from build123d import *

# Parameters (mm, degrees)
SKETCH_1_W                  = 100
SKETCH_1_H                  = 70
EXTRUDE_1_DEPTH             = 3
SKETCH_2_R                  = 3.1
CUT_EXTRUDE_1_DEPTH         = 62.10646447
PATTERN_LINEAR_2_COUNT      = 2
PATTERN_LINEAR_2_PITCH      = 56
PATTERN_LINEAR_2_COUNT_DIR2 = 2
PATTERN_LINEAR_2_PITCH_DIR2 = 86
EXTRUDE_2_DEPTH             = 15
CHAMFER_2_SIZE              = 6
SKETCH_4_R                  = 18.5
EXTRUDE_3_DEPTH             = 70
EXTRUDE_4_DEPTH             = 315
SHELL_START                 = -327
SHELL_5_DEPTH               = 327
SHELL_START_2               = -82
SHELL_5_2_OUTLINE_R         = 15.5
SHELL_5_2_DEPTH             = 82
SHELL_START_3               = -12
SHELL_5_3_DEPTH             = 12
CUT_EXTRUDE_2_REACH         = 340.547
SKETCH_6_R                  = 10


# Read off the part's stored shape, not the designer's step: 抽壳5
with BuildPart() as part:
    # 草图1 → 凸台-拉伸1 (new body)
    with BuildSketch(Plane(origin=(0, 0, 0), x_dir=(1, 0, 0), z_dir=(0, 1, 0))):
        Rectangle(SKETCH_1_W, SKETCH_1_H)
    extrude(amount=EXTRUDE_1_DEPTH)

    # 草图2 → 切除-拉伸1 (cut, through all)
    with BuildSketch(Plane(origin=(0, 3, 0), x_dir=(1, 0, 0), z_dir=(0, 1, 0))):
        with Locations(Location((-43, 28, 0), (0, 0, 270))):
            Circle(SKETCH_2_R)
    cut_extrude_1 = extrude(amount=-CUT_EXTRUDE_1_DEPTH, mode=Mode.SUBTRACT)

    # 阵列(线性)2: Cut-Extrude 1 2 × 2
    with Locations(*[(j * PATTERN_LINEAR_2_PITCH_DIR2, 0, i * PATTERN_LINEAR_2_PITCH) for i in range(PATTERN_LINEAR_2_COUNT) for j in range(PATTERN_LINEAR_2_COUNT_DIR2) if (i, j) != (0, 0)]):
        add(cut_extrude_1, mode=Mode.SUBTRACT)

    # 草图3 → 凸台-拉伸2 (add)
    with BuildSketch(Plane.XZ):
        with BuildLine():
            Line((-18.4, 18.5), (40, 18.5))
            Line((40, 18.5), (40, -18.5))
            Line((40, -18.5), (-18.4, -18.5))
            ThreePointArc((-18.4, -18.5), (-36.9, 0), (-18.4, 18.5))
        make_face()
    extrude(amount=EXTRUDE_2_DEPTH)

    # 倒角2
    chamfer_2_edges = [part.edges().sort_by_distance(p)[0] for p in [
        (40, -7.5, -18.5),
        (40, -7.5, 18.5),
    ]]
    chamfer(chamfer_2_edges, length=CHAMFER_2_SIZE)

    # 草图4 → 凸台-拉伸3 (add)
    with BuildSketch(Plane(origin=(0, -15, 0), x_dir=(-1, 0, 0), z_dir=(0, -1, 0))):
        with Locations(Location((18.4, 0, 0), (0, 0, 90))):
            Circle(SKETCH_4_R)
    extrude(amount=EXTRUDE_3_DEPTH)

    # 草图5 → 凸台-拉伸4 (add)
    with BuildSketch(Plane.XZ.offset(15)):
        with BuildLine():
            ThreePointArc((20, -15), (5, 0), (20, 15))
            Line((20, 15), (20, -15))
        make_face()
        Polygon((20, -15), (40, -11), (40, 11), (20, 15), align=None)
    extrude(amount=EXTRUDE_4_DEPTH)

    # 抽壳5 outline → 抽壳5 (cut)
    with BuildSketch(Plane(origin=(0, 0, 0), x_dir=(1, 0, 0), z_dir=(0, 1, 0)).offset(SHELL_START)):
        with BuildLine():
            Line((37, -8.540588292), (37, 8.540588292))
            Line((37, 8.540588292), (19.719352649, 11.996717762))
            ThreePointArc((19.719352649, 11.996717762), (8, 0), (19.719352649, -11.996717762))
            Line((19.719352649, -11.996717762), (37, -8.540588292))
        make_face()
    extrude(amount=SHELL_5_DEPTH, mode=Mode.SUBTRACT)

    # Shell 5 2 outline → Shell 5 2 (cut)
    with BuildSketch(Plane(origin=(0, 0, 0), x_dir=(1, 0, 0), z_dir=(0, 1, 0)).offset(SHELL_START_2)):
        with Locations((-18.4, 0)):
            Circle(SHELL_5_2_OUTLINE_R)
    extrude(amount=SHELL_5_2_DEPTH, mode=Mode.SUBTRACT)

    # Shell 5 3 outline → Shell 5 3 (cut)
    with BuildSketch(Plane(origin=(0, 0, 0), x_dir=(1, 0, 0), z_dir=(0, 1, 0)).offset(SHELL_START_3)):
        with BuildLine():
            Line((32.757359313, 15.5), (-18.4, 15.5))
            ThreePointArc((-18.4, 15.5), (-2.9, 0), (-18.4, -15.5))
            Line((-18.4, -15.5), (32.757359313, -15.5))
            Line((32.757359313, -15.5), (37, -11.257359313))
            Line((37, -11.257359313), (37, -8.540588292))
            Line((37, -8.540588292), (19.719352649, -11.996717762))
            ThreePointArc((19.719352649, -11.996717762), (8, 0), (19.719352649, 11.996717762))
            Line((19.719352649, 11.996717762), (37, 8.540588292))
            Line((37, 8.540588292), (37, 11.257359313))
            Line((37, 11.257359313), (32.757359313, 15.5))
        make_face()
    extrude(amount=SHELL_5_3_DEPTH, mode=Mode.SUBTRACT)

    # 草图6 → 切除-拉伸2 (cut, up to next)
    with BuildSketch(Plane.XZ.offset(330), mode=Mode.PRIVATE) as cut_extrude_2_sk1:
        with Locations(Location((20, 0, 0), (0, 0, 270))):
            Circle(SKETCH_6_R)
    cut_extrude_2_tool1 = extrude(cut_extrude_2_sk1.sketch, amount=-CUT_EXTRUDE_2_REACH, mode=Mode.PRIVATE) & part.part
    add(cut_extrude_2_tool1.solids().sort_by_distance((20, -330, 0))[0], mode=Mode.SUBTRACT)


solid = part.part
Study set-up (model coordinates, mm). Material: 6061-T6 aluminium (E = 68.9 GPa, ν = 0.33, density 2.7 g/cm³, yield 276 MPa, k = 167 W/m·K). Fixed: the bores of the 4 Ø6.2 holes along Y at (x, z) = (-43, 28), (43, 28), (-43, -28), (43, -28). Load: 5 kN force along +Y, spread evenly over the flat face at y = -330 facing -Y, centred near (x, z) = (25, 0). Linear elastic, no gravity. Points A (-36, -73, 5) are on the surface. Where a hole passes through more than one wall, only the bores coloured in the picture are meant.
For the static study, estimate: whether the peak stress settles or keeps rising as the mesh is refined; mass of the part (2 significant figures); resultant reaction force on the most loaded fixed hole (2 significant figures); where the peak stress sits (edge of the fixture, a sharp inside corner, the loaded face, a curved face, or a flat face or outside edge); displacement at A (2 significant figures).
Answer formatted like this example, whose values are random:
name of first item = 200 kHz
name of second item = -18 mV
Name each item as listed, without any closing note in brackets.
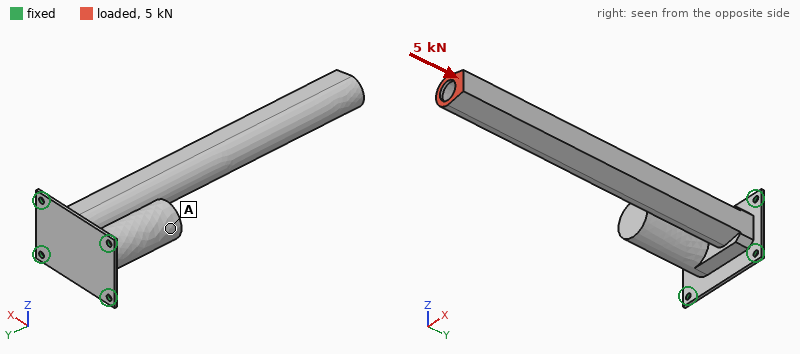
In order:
whether the peak stress settles or keeps rising as the mesh is refined = keeps rising
mass of the part = 410 g
resultant reaction force on the most loaded fixed hole = 2.2 kN
where the peak stress sits = edge of the fixture
displacement at A = 0.17 mm
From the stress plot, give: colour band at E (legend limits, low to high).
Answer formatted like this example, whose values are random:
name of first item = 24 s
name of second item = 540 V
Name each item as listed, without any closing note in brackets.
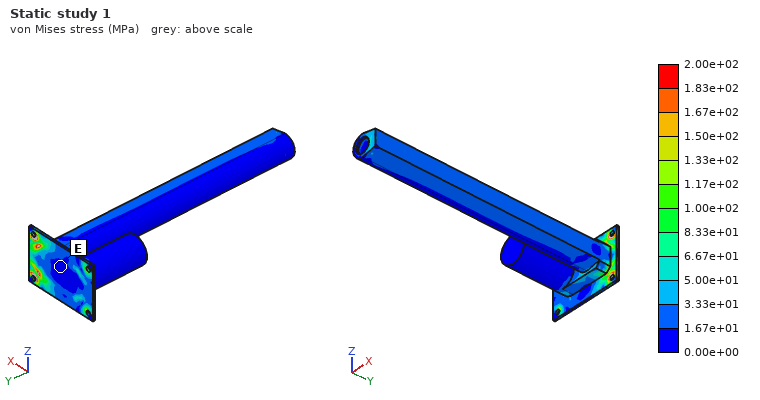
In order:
colour band at E = 0.00e+00 to 1.67e+01 MPa
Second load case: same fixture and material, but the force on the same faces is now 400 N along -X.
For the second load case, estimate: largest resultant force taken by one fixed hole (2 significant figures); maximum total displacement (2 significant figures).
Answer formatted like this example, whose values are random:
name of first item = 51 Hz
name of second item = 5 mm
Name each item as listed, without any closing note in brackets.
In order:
largest resultant force taken by one fixed hole = 1.2 kN
maximum total displacement = 3.7 mm
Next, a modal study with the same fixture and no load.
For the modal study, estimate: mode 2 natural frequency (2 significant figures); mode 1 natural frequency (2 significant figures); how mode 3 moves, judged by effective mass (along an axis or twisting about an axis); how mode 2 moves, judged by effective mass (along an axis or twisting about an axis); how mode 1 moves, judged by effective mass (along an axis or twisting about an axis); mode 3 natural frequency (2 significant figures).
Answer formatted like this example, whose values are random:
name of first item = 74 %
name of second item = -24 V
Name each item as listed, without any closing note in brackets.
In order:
mode 2 natural frequency = 180 Hz
mode 1 natural frequency = 150 Hz
how mode 3 moves, judged by effective mass = along Z
how mode 2 moves, judged by effective mass = along X
how mode 1 moves, judged by effective mass = along Z
mode 3 natural frequency = 1100 Hz
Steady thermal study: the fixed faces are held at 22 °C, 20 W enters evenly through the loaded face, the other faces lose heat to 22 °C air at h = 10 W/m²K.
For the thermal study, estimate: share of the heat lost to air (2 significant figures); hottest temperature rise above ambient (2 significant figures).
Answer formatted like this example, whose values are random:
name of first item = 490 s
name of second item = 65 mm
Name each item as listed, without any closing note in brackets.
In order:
share of the heat lost to air = 80 %
hottest temperature rise above ambient = 63 K
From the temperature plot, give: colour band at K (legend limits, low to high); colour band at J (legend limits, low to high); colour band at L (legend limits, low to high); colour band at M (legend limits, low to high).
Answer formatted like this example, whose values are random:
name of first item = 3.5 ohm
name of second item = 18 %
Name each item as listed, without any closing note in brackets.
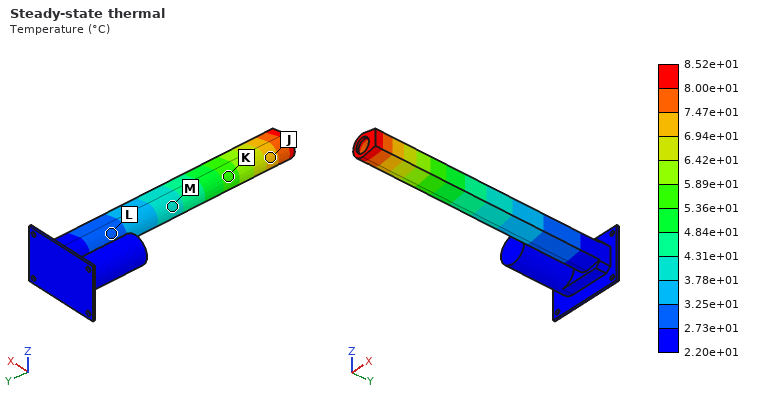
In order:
colour band at K = 5.36e+01 to 5.89e+01 °C
colour band at J = 6.94e+01 to 7.47e+01 °C
colour band at L = 2.73e+01 to 3.25e+01 °C
colour band at M = 3.78e+01 to 4.31e+01 °C
